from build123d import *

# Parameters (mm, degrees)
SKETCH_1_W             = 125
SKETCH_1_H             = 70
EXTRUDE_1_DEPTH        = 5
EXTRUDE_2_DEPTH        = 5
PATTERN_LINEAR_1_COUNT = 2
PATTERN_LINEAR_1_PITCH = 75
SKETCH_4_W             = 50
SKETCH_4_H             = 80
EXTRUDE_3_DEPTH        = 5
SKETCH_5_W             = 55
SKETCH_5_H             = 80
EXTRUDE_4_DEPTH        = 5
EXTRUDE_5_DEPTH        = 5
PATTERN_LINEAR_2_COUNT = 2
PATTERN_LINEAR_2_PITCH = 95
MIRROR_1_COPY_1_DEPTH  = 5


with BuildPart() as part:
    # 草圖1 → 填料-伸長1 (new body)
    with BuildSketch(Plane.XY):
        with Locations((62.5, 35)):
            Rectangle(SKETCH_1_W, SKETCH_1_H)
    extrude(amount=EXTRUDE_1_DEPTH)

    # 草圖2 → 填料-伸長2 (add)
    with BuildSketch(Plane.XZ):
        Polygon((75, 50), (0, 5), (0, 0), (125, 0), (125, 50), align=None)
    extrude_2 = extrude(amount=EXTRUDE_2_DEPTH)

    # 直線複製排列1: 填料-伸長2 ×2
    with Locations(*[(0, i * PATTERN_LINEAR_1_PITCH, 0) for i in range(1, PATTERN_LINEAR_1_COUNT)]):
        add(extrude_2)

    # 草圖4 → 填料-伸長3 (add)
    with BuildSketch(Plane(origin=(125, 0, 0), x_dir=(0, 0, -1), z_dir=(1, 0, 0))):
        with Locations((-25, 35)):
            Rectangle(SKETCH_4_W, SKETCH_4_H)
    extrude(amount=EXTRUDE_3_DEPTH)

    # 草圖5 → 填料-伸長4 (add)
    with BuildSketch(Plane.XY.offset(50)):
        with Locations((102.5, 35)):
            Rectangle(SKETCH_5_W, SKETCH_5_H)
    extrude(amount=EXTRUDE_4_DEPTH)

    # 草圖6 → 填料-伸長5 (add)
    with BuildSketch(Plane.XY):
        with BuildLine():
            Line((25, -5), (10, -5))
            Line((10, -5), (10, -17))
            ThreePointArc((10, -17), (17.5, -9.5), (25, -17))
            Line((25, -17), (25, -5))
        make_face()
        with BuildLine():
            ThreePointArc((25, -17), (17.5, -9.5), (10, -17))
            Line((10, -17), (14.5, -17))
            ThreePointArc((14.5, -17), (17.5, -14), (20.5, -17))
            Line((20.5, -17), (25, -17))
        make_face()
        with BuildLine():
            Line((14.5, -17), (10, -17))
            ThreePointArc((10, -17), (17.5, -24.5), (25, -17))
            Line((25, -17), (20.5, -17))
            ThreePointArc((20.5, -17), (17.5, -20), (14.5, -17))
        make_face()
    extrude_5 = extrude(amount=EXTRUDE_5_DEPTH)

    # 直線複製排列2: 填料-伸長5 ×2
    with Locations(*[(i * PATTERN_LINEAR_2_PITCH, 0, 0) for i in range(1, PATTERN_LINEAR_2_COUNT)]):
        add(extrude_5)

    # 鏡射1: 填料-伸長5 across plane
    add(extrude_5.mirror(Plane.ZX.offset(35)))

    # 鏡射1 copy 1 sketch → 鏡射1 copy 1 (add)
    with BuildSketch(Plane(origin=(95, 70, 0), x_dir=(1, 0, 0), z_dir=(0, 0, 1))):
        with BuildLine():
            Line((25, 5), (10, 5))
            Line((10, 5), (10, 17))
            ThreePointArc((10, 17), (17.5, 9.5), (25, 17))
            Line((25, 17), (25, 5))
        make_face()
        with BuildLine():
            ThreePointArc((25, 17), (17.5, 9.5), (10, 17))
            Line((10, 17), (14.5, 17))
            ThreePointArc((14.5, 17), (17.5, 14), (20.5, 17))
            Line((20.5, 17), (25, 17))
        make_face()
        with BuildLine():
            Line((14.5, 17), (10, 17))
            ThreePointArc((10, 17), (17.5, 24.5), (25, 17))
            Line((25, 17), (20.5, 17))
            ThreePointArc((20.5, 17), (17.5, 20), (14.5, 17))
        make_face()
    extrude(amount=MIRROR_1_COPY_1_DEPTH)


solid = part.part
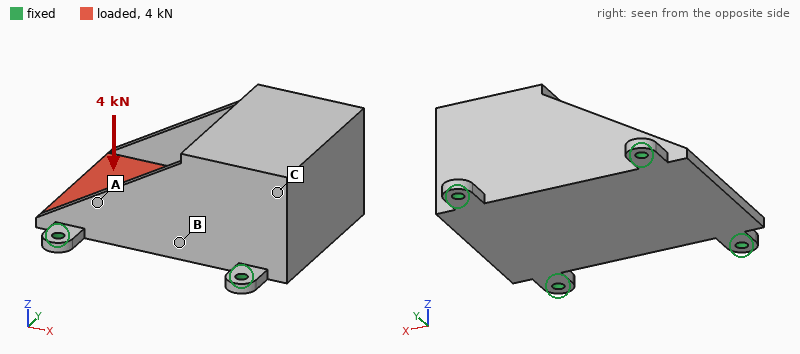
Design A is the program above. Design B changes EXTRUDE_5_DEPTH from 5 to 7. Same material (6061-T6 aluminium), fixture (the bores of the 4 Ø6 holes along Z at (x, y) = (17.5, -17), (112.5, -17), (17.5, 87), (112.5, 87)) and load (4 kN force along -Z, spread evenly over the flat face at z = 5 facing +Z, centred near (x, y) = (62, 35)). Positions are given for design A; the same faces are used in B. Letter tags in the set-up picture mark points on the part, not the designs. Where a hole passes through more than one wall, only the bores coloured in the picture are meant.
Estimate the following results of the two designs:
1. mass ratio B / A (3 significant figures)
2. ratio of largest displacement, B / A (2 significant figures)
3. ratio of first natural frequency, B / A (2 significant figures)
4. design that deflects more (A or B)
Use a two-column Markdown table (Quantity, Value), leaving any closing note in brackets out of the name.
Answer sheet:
| Quantity | Value |
|---|---|
| mass ratio B / A | 1.01 |
| ratio of largest displacement, B / A | 0.66 |
| ratio of first natural frequency, B / A | 1.2 |
| design that deflects more | A |
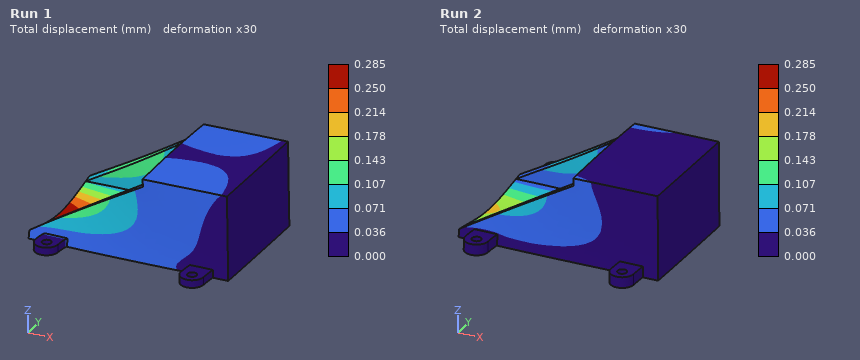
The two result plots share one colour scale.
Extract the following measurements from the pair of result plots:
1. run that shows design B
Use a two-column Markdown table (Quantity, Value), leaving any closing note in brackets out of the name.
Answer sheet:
| Quantity | Value |
|---|---|
| run that shows design B | Run 2 |
